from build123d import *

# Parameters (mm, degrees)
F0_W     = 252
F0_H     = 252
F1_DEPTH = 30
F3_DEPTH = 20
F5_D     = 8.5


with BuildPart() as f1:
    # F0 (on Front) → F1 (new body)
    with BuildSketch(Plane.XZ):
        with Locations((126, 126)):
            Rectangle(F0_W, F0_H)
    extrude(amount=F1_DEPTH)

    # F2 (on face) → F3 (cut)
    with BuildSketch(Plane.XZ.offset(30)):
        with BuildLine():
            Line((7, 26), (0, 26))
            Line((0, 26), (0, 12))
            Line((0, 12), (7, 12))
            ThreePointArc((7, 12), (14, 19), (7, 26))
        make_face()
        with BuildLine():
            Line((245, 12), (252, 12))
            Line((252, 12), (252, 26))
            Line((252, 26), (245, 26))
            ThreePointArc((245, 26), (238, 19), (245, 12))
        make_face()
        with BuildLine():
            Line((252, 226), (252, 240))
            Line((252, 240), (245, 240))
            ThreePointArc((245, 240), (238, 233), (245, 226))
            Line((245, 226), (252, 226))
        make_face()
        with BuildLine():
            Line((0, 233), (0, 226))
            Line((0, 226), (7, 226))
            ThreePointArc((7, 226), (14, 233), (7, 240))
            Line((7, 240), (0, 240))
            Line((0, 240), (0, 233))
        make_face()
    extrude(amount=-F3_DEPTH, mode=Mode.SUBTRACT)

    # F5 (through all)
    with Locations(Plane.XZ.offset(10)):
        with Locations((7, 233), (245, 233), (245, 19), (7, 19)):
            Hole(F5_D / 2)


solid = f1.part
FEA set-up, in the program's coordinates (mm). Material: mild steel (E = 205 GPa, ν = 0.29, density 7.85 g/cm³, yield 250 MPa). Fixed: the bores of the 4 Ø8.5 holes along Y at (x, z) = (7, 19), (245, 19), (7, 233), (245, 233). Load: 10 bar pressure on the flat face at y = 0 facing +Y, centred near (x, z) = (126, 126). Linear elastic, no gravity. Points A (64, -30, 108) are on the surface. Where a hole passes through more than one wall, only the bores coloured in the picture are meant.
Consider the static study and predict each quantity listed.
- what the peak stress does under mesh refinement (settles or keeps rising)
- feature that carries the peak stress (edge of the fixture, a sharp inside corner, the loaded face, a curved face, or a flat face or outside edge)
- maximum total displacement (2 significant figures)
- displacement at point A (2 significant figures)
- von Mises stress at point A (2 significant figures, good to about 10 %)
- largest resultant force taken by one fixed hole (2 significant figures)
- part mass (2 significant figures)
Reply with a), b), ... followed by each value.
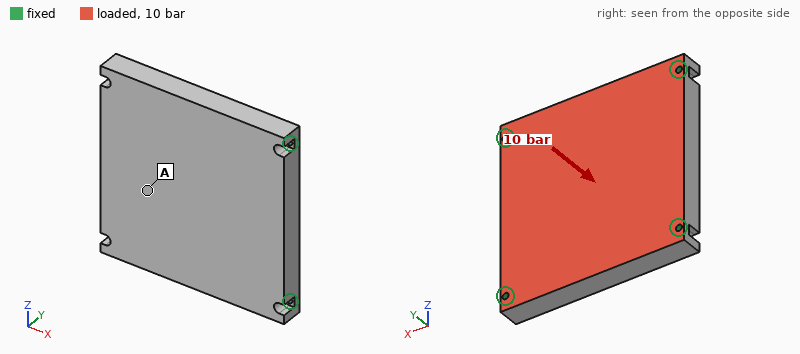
a) keeps rising
b) edge of the fixture
c) 90 µm
d) 75 µm
e) 27 MPa
f) 25 kN
g) 15 kg
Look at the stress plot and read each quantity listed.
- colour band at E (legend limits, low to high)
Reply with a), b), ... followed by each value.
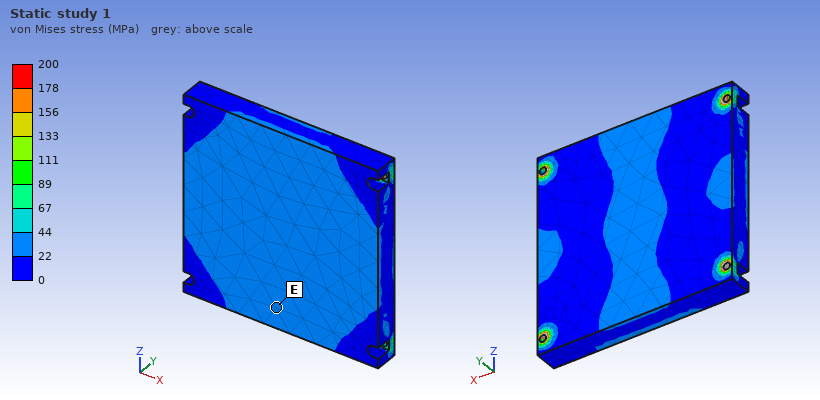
a) 22 to 44 MPa
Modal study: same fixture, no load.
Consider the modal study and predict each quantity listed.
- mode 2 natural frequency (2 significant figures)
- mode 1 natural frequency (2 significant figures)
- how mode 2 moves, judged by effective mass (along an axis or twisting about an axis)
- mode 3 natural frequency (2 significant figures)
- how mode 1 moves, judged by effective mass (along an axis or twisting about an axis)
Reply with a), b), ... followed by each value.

a) 2100 Hz
b) 1300 Hz
c) twisting about X
d) 2400 Hz
e) along Y
